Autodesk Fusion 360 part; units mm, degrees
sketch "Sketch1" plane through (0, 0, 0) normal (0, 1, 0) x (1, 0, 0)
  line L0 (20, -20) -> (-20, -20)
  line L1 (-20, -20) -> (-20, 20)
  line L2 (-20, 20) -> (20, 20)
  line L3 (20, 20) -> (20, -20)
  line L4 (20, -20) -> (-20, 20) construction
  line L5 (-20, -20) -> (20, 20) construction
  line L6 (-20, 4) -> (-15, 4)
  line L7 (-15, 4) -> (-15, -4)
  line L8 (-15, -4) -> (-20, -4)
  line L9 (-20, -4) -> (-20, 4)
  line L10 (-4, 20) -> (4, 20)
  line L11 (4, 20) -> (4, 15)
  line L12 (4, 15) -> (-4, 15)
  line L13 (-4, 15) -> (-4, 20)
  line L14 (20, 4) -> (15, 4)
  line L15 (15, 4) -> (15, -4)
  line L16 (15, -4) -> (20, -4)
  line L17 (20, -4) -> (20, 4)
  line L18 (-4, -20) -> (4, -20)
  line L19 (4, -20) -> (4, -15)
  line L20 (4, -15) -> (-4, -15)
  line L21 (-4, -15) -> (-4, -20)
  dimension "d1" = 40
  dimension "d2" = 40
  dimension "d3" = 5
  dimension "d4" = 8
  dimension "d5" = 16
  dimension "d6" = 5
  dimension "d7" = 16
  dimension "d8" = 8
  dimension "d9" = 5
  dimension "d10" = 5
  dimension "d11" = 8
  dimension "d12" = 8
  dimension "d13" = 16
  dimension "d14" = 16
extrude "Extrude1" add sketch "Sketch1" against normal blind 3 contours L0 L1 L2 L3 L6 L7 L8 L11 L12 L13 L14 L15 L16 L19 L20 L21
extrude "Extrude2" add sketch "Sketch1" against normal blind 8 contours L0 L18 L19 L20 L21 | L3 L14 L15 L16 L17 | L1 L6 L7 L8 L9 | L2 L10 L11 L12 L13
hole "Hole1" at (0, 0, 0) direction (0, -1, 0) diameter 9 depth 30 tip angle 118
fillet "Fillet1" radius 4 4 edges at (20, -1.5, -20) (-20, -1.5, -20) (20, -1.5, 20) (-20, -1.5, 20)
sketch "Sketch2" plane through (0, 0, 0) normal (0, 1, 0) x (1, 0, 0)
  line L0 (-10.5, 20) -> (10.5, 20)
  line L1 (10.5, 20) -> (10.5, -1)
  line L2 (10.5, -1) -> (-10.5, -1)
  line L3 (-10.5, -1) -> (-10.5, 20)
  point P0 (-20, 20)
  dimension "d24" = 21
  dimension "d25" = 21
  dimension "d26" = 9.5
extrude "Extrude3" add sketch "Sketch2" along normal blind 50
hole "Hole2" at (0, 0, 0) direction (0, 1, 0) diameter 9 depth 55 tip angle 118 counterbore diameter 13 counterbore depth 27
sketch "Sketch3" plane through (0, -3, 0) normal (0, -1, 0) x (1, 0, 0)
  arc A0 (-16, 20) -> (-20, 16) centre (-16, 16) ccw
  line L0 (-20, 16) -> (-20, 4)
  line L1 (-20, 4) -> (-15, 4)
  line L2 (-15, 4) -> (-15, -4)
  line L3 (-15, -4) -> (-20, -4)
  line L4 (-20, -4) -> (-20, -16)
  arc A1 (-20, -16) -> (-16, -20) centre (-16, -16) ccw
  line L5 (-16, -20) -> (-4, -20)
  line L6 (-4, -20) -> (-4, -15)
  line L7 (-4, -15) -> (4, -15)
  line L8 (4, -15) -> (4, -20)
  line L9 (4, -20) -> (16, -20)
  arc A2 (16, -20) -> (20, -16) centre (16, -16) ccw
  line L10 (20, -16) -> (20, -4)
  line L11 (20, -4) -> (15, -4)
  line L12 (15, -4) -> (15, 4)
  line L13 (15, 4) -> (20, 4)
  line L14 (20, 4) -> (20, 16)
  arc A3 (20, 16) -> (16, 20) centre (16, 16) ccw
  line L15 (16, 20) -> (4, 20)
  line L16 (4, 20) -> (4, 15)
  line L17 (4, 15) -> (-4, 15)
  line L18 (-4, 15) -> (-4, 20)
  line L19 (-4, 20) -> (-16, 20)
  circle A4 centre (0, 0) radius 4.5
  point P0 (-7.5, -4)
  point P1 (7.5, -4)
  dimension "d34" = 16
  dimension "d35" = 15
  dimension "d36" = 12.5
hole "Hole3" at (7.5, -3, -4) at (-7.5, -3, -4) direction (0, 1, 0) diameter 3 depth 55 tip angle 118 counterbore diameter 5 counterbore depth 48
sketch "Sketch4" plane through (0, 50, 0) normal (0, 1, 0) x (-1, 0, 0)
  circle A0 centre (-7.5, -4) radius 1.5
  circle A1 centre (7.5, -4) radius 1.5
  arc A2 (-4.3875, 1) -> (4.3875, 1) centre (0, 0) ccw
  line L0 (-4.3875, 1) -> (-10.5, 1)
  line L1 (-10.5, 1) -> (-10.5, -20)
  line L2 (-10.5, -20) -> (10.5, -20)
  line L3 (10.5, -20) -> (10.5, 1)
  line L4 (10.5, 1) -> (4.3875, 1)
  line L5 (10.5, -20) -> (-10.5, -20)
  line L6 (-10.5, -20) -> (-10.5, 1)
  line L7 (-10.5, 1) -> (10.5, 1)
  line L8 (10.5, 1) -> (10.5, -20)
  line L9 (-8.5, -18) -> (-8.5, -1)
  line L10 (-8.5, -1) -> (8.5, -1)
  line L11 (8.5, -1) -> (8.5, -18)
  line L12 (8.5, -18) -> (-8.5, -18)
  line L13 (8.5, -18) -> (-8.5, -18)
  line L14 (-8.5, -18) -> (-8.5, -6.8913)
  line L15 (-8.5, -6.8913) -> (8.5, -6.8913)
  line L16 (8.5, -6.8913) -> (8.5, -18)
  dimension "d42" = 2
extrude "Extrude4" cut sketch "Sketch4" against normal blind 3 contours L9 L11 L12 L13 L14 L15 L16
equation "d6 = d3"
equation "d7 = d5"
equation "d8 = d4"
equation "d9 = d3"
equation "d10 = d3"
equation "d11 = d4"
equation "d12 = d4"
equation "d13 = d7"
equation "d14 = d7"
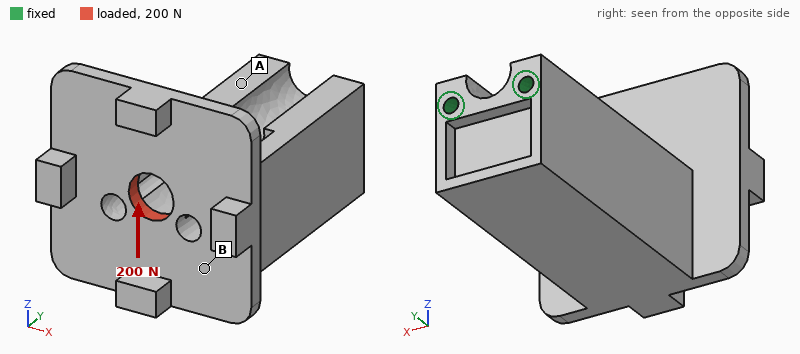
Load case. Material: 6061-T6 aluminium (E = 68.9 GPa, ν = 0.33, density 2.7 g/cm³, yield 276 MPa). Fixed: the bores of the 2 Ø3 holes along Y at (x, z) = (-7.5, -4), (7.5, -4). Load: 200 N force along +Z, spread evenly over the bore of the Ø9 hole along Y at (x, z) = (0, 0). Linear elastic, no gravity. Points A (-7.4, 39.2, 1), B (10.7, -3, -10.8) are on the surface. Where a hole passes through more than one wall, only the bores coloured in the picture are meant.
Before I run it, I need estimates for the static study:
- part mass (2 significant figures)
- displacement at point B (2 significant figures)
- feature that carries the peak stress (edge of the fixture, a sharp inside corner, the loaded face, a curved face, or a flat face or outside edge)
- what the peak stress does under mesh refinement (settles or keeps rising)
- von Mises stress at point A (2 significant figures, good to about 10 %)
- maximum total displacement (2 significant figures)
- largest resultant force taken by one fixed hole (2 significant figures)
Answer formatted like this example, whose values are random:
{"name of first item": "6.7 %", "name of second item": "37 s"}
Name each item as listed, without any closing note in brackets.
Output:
{"part mass": "59 g", "displacement at point B": "0.099 mm", "feature that carries the peak stress": "edge of the fixture", "what the peak stress does under mesh refinement": "keeps rising", "von Mises stress at point A": "18 MPa", "maximum total displacement": "0.12 mm", "largest resultant force taken by one fixed hole": "100 N"}
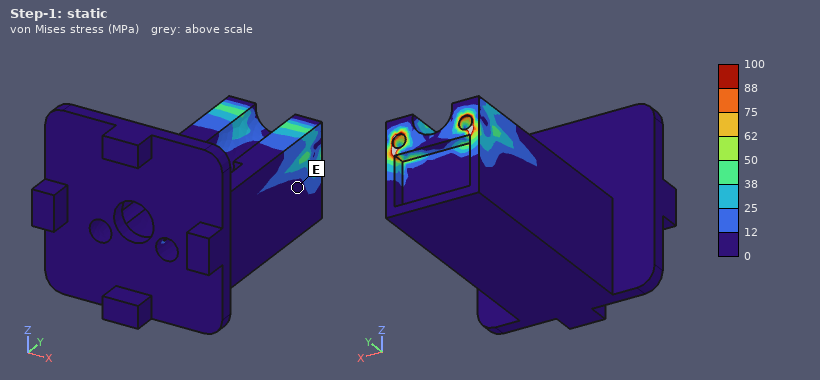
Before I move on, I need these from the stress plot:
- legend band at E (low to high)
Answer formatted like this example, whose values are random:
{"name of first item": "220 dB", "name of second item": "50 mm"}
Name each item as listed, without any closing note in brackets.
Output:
{"legend band at E": "0 to 12 MPa"}
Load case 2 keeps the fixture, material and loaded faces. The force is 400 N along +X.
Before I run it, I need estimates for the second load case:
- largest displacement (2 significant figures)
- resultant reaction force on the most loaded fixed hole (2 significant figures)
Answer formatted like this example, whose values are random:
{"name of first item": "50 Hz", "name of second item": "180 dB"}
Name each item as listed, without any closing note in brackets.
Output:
{"largest displacement": "91 µm", "resultant reaction force on the most loaded fixed hole": "1.2 kN"}
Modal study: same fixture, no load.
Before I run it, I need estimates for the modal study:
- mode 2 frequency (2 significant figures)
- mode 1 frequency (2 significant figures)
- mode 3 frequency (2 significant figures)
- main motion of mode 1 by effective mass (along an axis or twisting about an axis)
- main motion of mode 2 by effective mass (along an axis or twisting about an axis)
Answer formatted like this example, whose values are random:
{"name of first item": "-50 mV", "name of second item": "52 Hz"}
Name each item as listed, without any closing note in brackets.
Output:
{"mode 2 frequency": "2600 Hz", "mode 1 frequency": "1300 Hz", "mode 3 frequency": "3900 Hz", "main motion of mode 1 by effective mass": "along Z", "main motion of mode 2 by effective mass": "along X"}
